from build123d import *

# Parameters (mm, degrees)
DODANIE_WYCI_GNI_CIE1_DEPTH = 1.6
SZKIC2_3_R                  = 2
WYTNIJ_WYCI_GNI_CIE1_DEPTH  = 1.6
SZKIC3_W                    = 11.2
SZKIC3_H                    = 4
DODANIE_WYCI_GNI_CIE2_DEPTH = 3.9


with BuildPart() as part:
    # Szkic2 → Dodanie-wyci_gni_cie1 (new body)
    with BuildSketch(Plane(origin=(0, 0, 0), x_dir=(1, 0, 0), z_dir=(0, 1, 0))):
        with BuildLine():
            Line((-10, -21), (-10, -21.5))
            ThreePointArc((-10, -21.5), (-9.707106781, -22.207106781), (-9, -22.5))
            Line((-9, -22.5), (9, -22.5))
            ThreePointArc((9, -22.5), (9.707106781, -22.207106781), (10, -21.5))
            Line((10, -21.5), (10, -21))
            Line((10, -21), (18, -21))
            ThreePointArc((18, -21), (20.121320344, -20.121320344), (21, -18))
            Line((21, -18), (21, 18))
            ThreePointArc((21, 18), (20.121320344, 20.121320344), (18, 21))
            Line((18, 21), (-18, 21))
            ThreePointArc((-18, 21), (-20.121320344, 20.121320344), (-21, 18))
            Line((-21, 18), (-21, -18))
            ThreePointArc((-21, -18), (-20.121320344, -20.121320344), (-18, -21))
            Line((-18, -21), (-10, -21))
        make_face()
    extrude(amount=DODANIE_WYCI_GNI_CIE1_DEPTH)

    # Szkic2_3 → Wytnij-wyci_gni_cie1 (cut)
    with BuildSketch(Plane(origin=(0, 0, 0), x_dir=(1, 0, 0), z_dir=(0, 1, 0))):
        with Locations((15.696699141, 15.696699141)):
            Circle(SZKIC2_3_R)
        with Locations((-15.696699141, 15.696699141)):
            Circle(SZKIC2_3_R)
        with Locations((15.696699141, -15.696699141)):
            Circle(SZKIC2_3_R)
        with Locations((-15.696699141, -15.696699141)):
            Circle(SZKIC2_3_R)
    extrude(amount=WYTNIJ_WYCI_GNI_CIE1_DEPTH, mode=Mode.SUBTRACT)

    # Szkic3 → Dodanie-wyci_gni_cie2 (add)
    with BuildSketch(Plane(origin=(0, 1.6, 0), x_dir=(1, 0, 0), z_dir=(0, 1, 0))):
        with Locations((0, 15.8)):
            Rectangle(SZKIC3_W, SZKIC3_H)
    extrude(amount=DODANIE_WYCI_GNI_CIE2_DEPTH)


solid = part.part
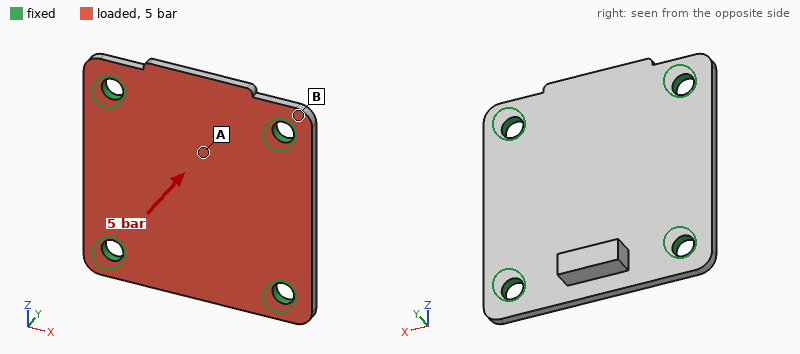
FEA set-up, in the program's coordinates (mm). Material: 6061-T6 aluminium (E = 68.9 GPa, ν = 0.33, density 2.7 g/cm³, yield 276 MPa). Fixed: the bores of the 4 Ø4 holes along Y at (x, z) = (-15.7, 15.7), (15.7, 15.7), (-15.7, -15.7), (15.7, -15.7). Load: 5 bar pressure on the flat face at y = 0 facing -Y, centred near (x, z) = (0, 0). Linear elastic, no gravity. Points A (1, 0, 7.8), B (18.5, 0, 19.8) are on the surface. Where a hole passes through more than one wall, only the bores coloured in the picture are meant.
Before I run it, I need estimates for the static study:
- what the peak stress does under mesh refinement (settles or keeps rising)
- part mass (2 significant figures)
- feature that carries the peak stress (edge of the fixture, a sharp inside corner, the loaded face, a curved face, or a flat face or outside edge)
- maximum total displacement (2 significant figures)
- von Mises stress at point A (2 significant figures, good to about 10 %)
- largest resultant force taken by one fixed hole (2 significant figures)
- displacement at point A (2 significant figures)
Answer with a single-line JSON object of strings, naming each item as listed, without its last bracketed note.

{"what the peak stress does under mesh refinement": "keeps rising", "part mass": "8.0 g", "feature that carries the peak stress": "edge of the fixture", "maximum total displacement": "91 µm", "von Mises stress at point A": "43 MPa", "largest resultant force taken by one fixed hole": "220 N", "displacement at point A": "78 µm"}
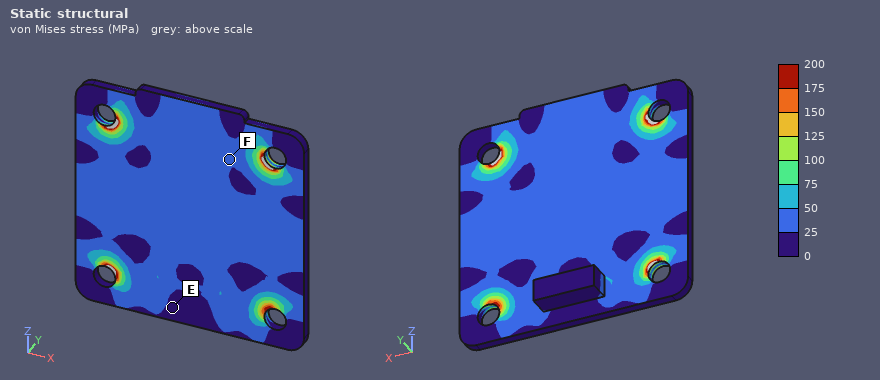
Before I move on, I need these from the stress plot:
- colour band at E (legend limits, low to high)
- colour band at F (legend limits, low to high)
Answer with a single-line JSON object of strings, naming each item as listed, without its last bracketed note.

{"colour band at E": "0 to 25 MPa", "colour band at F": "25 to 50 MPa"}
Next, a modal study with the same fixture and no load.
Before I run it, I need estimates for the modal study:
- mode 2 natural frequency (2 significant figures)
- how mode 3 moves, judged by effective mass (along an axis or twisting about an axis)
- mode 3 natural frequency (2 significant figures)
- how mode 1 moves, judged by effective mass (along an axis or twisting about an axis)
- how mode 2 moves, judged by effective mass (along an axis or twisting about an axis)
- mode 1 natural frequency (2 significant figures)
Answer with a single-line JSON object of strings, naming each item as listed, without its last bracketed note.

{"mode 2 natural frequency": "10000 Hz", "how mode 3 moves, judged by effective mass": "twisting about Z", "mode 3 natural frequency": "11 kHz", "how mode 1 moves, judged by effective mass": "along Y", "how mode 2 moves, judged by effective mass": "twisting about X", "mode 1 natural frequency": "6900 Hz"}
